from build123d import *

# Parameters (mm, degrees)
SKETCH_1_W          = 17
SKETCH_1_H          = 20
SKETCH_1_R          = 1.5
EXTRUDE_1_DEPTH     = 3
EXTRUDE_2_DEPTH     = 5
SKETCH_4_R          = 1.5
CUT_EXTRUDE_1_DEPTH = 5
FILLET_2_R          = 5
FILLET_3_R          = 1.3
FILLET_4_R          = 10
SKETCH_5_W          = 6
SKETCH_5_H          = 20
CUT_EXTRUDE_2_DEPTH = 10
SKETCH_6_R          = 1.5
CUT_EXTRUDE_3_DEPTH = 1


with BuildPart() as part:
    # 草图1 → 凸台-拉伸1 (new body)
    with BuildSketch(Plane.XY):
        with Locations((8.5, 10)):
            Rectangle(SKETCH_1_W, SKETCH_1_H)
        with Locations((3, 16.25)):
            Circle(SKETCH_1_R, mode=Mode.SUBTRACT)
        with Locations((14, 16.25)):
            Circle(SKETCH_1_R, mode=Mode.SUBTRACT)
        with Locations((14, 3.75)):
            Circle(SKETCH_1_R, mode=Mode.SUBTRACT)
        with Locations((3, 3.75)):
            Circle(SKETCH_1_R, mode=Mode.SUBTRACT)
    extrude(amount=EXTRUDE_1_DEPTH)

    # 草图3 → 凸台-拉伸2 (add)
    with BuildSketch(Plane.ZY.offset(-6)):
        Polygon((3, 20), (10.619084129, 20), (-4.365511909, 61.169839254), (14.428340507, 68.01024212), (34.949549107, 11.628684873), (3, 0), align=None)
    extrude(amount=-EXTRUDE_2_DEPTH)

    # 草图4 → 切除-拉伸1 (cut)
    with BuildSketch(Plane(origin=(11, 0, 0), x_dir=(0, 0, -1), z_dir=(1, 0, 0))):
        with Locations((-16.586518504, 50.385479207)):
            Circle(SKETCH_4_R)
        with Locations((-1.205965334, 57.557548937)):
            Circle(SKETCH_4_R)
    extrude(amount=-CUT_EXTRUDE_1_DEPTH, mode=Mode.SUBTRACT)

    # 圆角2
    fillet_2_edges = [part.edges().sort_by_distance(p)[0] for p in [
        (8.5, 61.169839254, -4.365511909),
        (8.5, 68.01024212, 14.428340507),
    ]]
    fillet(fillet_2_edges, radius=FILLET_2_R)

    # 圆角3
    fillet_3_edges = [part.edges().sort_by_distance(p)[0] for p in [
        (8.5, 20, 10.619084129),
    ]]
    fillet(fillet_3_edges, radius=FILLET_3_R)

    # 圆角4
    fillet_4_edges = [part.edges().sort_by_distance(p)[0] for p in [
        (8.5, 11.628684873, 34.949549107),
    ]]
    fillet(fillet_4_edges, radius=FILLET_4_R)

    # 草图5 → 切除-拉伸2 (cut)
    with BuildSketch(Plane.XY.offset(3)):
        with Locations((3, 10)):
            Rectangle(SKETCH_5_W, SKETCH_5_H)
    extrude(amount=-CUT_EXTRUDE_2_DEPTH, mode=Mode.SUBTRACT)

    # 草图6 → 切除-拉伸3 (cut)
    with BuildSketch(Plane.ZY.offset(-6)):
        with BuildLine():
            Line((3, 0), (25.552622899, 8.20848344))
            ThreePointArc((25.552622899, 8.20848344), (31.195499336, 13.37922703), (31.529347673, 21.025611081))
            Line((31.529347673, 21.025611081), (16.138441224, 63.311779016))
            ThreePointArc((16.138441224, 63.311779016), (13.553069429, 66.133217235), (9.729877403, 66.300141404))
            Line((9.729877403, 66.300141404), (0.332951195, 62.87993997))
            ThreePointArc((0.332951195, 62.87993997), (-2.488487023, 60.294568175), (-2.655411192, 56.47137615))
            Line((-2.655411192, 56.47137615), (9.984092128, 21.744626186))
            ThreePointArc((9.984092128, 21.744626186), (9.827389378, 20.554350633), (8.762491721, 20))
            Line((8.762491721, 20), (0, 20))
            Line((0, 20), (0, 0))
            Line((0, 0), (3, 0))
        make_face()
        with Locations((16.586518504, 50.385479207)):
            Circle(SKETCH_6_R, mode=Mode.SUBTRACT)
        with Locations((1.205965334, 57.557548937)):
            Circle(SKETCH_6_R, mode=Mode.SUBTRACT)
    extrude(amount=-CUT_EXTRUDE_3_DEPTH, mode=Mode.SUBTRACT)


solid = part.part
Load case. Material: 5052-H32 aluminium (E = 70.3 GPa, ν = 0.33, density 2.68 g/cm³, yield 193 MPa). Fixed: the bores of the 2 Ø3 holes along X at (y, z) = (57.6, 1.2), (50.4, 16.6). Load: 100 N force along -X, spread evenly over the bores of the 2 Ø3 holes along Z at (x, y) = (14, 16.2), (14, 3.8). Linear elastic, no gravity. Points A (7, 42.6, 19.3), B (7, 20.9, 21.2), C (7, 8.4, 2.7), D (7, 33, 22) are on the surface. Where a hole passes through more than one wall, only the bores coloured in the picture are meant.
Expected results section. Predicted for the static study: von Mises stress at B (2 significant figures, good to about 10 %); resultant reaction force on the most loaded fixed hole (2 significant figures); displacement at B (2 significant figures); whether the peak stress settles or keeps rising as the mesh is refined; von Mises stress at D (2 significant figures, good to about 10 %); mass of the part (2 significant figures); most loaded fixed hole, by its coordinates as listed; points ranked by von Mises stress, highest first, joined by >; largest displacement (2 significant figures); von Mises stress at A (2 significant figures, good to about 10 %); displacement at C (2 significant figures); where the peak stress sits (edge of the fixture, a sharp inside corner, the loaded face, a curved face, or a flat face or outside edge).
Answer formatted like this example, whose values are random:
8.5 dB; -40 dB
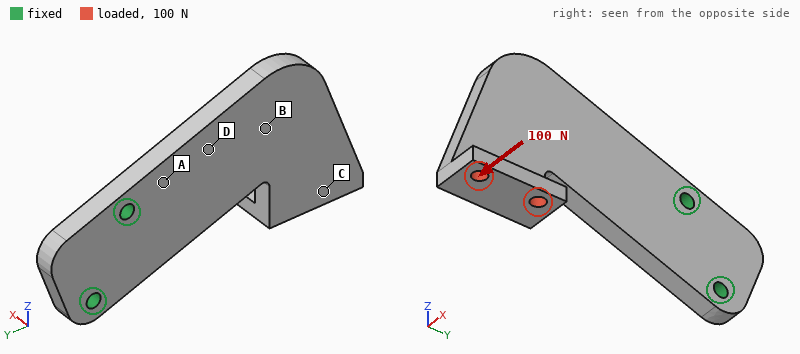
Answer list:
27 MPa; 130 N; 0.17 mm; keeps rising; 44 MPa; 16 g; (50.4, 16.6); A > D > B > C; 0.54 mm; 66 MPa; 0.41 mm; edge of the fixture
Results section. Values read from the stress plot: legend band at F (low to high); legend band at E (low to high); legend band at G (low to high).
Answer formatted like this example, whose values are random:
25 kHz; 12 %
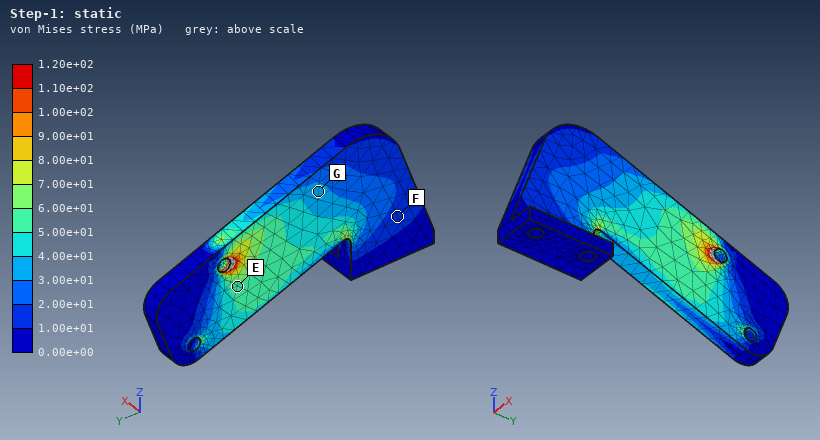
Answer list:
1.00e+01 to 2.00e+01 MPa; 5.00e+01 to 6.00e+01 MPa; 3.00e+01 to 4.00e+01 MPa
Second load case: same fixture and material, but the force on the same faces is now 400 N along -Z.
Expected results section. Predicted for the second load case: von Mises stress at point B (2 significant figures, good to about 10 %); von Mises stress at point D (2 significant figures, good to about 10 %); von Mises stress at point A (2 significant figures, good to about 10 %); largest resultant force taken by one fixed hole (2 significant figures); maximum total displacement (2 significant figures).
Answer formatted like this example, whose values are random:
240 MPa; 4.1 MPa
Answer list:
18 MPa; 34 MPa; 49 MPa; 1.0 kN; 0.24 mm
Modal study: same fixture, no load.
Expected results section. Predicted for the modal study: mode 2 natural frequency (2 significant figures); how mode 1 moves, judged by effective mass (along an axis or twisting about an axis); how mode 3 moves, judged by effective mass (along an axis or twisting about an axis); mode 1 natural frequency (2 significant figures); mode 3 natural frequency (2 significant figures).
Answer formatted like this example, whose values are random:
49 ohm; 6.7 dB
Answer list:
3300 Hz; along X; along Z; 1100 Hz; 4600 Hz
